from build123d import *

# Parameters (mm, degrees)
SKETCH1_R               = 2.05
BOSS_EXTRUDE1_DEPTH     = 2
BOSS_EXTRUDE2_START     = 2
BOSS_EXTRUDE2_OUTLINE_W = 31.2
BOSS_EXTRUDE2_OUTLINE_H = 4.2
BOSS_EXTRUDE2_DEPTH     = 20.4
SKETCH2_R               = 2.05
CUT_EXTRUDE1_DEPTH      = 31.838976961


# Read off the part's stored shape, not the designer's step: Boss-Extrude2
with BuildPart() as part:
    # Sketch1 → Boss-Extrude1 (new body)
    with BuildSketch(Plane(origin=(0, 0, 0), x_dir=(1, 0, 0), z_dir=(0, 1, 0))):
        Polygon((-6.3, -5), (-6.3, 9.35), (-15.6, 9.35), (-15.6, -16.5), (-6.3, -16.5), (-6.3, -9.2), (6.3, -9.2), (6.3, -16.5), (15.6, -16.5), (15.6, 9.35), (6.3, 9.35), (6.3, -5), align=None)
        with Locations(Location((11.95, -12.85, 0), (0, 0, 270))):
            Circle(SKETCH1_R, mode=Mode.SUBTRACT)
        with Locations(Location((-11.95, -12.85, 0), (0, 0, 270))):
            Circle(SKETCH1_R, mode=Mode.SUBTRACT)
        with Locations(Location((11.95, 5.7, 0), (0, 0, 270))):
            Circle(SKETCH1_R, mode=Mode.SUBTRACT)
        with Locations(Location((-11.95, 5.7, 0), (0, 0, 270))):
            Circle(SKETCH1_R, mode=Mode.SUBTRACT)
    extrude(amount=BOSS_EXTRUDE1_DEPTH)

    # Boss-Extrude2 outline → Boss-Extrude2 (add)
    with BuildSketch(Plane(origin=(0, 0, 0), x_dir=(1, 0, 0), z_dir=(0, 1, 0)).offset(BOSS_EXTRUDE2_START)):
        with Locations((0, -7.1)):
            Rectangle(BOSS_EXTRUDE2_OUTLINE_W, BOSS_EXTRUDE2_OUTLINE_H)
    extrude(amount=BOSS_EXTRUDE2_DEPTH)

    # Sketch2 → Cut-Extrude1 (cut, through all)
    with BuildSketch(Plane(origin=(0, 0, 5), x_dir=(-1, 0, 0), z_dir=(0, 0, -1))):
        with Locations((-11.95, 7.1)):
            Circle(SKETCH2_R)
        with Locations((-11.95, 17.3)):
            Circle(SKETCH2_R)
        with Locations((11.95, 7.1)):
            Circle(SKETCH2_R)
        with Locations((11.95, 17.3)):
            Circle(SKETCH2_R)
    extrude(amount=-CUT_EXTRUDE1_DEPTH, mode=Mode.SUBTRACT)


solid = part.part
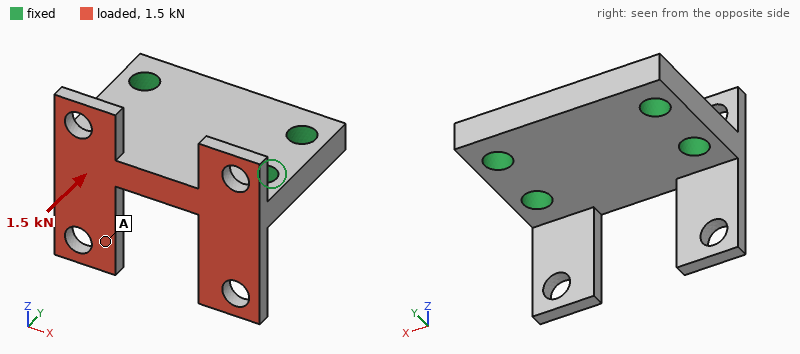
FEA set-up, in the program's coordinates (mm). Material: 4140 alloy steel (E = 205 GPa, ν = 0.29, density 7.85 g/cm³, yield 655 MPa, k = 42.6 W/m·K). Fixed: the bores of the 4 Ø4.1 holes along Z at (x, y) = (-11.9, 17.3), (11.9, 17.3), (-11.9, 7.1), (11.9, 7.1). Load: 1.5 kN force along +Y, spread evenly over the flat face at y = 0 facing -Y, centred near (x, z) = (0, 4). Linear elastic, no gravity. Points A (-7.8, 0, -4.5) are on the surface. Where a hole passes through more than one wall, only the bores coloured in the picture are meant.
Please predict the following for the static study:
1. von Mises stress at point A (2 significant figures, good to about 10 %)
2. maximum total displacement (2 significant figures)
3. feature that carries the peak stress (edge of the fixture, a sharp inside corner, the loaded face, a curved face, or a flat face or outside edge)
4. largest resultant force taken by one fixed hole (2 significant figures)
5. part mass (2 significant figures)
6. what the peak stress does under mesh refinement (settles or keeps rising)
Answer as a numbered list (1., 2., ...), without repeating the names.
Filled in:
1. 68 MPa
2. 0.14 mm
3. a sharp inside corner
4. 660 N
5. 27 g
6. keeps rising
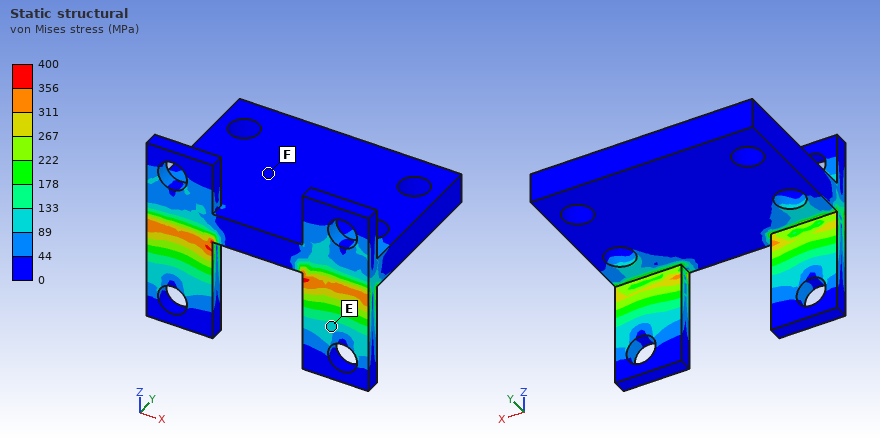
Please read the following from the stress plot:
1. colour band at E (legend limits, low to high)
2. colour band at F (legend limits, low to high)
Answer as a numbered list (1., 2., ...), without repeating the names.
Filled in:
1. 89 to 133 MPa
2. 0 to 44 MPa
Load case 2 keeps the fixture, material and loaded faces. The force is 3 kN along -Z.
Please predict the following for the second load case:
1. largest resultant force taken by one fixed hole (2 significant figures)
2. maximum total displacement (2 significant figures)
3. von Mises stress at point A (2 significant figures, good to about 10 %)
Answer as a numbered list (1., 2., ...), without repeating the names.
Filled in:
1. 1.7 kN
2. 84 µm
3. 67 MPa
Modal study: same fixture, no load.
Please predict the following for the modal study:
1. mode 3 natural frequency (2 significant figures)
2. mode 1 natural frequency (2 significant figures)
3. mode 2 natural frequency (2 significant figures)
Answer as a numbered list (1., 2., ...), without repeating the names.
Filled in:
1. 17 kHz
2. 7300 Hz
3. 7300 Hz
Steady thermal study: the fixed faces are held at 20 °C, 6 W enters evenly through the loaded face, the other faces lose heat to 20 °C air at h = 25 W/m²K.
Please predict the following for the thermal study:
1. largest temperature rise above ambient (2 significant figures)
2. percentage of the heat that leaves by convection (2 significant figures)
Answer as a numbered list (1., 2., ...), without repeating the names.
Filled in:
1. 22 K
2. 5.1 %
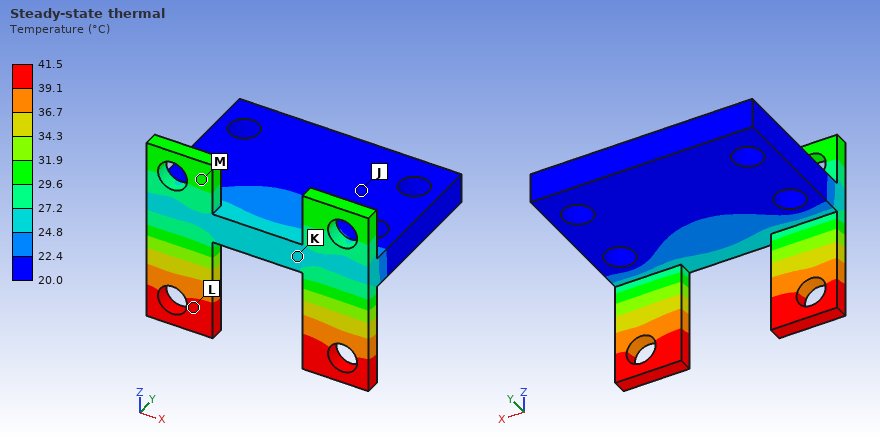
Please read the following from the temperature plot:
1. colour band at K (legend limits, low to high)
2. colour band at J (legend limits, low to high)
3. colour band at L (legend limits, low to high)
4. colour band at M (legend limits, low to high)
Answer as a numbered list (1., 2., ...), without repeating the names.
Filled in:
1. 24.8 to 27.2 °C
2. 20.0 to 22.4 °C
3. 39.1 to 41.5 °C
4. 29.6 to 31.9 °C
